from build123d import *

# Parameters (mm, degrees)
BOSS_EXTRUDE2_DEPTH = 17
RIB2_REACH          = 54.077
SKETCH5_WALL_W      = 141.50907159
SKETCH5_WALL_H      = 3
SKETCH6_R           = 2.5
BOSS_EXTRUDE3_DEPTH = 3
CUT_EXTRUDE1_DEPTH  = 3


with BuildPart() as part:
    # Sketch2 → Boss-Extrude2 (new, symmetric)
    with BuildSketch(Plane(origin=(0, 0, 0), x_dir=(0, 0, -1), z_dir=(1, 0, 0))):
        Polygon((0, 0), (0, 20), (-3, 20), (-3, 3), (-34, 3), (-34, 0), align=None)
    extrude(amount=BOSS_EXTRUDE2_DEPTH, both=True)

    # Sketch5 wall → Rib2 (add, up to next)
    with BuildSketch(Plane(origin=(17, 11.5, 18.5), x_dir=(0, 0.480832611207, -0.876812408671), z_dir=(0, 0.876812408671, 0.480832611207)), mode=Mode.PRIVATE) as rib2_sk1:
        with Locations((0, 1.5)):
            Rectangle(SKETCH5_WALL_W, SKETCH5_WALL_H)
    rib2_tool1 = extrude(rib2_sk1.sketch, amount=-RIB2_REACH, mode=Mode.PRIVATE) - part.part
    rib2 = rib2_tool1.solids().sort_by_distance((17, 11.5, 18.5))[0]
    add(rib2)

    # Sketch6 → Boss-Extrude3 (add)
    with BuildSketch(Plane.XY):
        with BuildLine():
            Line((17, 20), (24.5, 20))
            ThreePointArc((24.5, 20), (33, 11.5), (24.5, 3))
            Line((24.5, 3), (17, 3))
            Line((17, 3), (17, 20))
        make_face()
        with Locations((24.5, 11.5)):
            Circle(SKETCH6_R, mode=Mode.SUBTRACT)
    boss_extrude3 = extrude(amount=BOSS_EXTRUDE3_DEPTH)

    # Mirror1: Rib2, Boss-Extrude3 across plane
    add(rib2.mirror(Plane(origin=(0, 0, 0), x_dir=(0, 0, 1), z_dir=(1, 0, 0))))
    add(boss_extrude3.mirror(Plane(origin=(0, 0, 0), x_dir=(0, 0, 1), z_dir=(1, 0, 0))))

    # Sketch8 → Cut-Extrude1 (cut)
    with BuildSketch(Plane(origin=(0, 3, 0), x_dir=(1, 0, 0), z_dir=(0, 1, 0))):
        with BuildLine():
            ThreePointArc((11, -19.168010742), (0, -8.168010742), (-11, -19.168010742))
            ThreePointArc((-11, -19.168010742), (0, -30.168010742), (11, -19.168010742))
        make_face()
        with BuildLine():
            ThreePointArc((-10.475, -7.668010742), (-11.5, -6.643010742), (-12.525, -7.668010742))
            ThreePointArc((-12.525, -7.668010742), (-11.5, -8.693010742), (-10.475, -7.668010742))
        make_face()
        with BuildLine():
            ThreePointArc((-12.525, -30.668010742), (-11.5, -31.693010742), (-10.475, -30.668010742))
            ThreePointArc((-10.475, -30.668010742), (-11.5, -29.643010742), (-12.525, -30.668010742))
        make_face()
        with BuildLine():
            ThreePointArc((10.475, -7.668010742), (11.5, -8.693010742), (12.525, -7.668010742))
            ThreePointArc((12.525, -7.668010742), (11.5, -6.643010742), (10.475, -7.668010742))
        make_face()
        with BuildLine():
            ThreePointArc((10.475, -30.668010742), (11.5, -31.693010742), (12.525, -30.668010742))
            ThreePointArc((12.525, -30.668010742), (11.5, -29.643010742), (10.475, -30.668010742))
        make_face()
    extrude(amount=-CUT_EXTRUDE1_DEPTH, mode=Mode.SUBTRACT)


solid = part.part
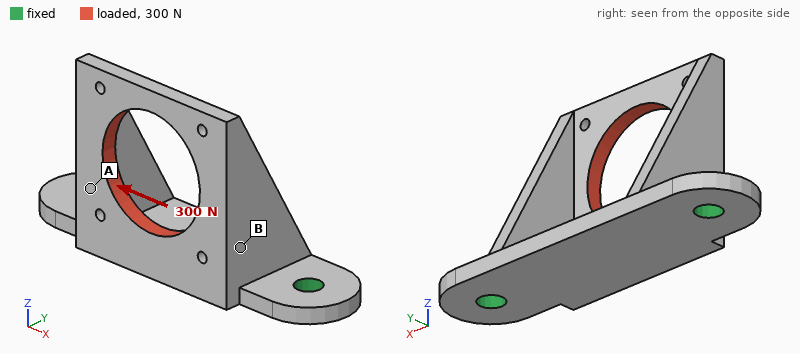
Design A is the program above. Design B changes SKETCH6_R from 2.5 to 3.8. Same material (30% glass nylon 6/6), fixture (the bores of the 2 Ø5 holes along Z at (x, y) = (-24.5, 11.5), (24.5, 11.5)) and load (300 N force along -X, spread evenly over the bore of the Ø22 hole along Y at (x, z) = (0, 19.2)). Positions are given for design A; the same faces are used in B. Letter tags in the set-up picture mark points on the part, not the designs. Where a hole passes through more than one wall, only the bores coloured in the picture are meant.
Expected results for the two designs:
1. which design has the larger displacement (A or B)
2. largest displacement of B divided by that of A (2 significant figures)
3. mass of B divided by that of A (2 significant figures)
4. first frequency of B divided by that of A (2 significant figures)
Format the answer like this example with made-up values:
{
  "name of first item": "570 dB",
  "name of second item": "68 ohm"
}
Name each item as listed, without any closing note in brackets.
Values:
{
  "which design has the larger displacement": "A",
  "largest displacement of B divided by that of A": "0.86",
  "mass of B divided by that of A": "0.98",
  "first frequency of B divided by that of A": "1.2"
}
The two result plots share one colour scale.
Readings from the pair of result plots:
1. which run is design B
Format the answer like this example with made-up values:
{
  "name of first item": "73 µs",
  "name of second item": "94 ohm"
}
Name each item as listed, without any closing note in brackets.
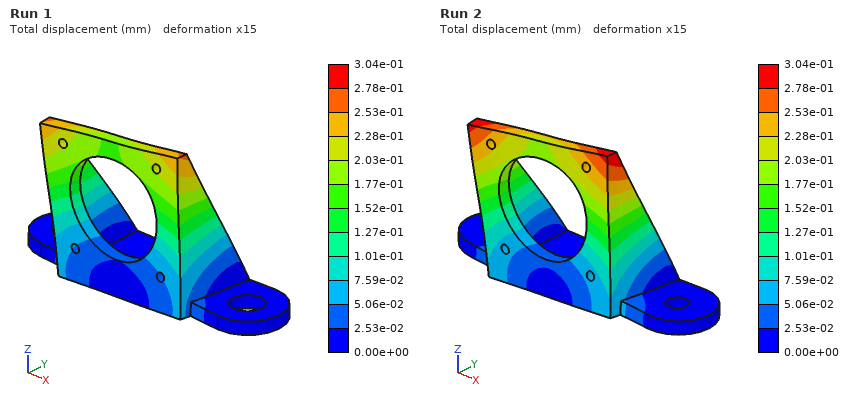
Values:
{
  "which run is design B": "Run 1"
}
